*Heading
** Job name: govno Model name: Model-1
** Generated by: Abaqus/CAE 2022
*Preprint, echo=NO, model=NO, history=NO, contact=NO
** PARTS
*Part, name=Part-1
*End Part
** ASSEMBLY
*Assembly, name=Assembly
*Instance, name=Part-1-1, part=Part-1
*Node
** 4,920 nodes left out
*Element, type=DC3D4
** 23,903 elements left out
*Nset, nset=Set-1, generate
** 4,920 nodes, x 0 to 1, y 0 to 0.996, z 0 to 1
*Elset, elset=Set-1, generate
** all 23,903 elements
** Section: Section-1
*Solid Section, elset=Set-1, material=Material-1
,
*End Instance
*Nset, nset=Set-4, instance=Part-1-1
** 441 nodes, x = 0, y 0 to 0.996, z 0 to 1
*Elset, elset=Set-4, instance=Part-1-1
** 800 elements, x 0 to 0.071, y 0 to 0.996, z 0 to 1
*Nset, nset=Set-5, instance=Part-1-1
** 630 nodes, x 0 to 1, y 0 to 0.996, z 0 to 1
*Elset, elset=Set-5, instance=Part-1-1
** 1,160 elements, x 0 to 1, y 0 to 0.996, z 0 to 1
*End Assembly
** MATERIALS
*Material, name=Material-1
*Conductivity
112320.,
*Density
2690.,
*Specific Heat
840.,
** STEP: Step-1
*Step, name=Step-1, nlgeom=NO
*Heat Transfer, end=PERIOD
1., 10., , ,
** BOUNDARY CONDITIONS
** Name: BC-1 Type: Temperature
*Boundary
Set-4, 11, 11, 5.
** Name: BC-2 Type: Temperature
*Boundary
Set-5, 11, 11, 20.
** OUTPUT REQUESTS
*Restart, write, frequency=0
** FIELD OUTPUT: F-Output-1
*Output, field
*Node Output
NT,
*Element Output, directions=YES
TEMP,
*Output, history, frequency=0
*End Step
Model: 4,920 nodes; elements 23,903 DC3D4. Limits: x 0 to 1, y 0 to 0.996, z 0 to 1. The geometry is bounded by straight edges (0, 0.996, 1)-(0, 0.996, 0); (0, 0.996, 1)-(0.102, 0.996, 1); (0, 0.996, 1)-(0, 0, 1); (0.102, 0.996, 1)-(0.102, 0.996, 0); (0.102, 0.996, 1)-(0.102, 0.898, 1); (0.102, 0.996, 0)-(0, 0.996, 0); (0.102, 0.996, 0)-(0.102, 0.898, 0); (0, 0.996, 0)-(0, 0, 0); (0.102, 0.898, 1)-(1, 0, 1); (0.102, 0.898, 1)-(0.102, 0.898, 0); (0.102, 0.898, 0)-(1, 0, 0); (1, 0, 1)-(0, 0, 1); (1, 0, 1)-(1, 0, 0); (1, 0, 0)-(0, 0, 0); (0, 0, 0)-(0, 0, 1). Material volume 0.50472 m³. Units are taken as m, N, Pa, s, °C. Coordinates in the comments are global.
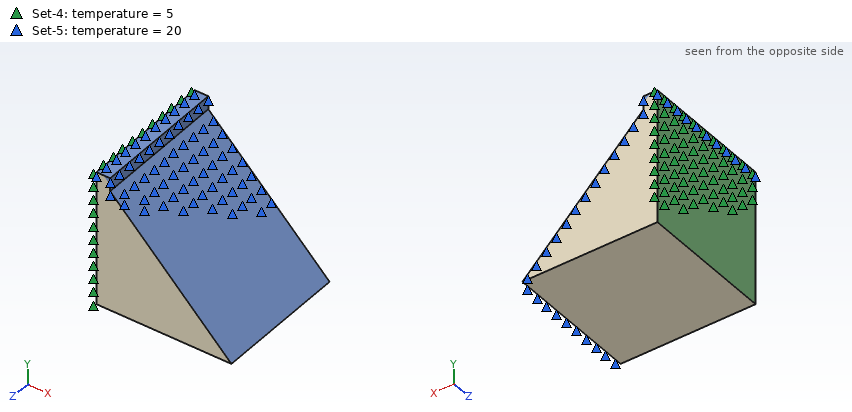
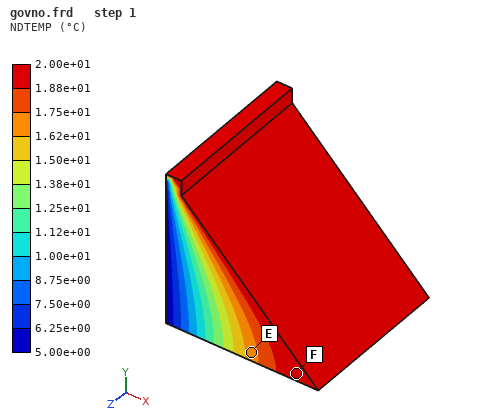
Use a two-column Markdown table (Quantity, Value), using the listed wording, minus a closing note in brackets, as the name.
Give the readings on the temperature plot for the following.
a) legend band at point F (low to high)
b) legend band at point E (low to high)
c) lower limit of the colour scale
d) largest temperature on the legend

| Quantity | Value |
|---|---|
| legend band at point F | 1.88e+01 to 2.00e+01 °C |
| legend band at point E | 1.62e+01 to 1.75e+01 °C |
| lower limit of the colour scale | 5.00e+00 °C |
| largest temperature on the legend | 2.00e+01 °C |
